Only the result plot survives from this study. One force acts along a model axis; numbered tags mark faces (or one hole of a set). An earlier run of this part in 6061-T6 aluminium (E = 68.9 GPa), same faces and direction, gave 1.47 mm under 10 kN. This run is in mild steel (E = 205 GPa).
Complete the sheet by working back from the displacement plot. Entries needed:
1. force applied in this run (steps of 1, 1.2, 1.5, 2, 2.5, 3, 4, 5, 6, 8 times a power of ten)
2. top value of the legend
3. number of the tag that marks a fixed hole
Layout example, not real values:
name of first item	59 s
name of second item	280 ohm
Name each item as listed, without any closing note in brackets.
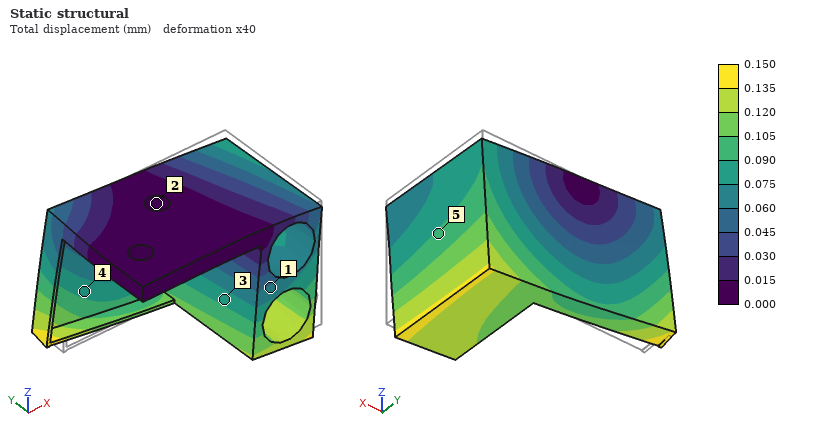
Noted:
force applied in this run	3 kN
top value of the legend	0.150 mm
number of the tag that marks a fixed hole	2
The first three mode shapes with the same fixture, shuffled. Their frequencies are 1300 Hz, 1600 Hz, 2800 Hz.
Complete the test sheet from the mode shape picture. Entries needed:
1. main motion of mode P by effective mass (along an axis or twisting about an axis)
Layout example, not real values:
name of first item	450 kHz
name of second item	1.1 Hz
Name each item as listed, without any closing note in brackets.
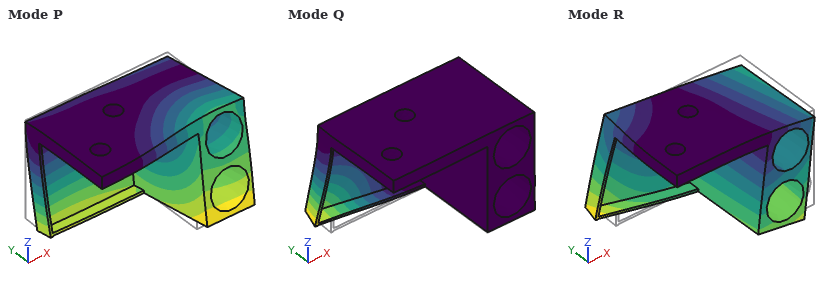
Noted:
main motion of mode P by effective mass	along Y
